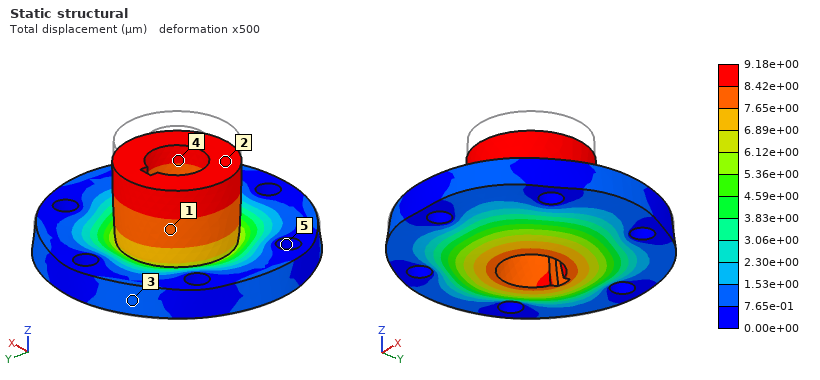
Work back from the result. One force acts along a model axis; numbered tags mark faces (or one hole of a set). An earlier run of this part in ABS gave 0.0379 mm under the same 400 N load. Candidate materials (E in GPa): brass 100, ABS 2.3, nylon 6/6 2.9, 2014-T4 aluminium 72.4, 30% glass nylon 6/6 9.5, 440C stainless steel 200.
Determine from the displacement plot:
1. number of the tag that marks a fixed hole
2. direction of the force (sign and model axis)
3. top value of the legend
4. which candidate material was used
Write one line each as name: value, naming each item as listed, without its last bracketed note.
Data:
number of the tag that marks a fixed hole: 5
direction of the force: -Z
top value of the legend: 9.18e+00 µm
which candidate material was used: 30% glass nylon 6/6
